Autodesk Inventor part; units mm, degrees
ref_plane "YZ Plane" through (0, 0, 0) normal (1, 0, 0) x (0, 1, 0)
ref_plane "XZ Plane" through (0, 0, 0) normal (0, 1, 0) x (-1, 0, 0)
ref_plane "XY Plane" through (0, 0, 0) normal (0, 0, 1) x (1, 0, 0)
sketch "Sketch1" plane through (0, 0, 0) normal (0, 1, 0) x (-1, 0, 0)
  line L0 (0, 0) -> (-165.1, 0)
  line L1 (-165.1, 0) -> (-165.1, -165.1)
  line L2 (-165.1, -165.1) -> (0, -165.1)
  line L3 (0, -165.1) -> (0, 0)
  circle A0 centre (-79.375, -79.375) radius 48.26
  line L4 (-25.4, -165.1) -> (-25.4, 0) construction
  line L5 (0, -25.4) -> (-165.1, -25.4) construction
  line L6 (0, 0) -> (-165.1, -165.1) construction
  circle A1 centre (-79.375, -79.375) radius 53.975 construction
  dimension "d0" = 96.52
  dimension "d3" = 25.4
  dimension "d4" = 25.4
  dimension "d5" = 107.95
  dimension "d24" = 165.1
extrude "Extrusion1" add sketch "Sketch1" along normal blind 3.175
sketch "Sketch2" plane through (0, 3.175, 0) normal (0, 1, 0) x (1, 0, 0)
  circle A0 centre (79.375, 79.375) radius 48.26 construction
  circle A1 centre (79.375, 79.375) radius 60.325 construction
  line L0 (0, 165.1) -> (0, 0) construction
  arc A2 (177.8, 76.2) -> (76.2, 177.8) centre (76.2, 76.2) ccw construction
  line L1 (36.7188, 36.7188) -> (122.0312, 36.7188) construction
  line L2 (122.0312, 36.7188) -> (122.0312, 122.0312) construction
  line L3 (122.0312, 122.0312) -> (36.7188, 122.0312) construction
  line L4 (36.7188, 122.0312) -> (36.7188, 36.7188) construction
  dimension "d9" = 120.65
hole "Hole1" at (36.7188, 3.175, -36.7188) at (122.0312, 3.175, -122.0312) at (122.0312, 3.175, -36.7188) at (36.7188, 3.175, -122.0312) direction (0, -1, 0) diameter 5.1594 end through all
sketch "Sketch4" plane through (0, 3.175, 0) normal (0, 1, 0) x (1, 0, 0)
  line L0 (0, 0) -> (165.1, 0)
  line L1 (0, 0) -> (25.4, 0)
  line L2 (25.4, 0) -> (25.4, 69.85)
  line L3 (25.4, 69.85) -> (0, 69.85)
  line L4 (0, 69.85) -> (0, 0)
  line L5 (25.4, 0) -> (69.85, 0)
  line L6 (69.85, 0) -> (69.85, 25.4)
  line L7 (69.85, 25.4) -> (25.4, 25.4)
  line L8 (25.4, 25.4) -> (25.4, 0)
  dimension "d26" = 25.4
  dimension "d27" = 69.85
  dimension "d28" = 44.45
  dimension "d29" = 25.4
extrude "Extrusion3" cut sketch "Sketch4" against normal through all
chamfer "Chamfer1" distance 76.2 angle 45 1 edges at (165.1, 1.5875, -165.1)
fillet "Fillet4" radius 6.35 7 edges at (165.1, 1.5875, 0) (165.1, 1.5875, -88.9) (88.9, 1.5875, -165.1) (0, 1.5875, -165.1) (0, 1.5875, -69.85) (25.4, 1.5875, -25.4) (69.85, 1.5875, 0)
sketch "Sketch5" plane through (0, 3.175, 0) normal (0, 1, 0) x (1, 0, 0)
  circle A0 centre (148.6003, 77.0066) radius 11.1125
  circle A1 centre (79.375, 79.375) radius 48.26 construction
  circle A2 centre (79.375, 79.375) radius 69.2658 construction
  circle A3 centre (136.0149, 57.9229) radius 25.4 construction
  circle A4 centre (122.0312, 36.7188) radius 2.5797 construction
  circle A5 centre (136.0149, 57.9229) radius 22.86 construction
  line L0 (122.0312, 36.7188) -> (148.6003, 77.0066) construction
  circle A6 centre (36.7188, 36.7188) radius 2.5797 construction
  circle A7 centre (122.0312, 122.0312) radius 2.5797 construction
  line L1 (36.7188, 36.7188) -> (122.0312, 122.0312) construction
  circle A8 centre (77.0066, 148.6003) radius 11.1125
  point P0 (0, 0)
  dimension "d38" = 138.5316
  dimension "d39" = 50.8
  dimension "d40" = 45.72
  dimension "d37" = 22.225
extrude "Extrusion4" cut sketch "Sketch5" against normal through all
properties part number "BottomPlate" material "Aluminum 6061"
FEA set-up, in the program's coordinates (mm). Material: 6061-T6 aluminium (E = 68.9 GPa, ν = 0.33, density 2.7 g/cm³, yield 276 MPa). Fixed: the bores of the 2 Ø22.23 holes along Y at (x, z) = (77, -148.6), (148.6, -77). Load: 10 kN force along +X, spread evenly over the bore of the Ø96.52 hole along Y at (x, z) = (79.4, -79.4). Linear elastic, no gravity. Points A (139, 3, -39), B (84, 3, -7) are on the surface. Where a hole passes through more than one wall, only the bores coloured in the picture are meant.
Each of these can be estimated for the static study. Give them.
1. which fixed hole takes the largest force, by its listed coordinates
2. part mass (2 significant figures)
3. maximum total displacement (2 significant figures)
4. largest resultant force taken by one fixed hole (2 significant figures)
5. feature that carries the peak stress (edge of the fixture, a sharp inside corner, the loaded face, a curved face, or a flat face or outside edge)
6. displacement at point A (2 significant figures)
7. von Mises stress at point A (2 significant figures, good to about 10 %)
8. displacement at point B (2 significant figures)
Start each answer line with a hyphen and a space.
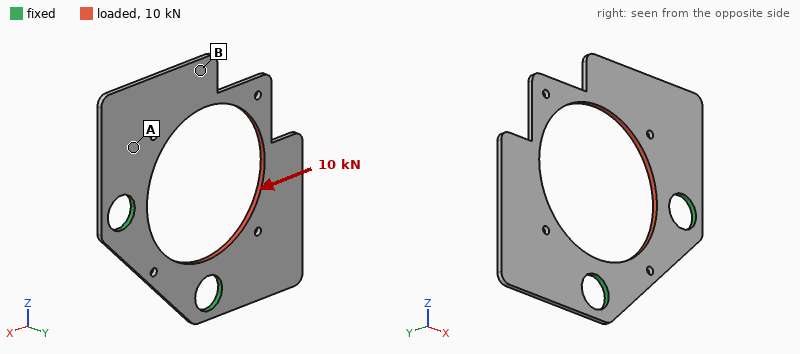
- (148.6, -77)
- 110 g
- 0.44 mm
- 5.6 kN
- edge of the fixture
- 0.12 mm
- 53 MPa
- 0.35 mm
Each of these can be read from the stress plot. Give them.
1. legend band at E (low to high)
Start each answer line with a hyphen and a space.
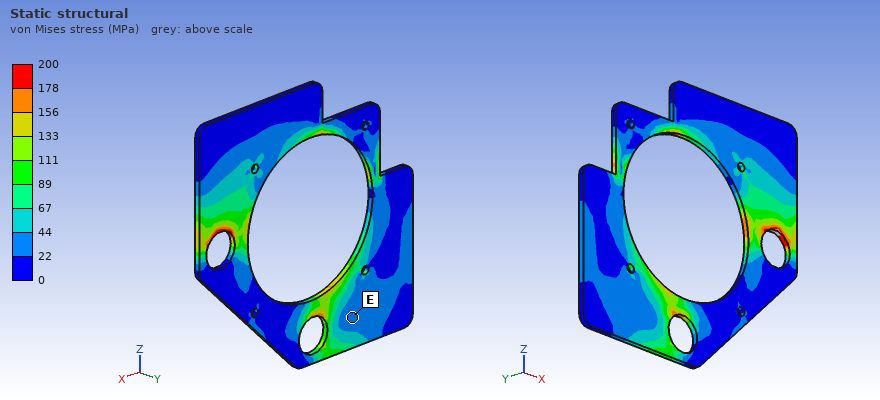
- 22 to 44 MPa
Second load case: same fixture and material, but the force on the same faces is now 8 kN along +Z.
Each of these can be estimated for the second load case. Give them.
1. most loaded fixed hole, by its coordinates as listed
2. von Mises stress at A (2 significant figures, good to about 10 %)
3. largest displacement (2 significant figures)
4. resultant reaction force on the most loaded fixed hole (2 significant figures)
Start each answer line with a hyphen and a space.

- (77, -148.6)
- 23 MPa
- 0.35 mm
- 4.5 kN
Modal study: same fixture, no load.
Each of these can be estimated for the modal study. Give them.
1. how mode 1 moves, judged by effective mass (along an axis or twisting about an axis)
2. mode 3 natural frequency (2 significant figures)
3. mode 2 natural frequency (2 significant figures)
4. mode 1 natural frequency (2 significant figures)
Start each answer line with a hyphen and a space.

- along Y
- 620 Hz
- 380 Hz
- 250 Hz
